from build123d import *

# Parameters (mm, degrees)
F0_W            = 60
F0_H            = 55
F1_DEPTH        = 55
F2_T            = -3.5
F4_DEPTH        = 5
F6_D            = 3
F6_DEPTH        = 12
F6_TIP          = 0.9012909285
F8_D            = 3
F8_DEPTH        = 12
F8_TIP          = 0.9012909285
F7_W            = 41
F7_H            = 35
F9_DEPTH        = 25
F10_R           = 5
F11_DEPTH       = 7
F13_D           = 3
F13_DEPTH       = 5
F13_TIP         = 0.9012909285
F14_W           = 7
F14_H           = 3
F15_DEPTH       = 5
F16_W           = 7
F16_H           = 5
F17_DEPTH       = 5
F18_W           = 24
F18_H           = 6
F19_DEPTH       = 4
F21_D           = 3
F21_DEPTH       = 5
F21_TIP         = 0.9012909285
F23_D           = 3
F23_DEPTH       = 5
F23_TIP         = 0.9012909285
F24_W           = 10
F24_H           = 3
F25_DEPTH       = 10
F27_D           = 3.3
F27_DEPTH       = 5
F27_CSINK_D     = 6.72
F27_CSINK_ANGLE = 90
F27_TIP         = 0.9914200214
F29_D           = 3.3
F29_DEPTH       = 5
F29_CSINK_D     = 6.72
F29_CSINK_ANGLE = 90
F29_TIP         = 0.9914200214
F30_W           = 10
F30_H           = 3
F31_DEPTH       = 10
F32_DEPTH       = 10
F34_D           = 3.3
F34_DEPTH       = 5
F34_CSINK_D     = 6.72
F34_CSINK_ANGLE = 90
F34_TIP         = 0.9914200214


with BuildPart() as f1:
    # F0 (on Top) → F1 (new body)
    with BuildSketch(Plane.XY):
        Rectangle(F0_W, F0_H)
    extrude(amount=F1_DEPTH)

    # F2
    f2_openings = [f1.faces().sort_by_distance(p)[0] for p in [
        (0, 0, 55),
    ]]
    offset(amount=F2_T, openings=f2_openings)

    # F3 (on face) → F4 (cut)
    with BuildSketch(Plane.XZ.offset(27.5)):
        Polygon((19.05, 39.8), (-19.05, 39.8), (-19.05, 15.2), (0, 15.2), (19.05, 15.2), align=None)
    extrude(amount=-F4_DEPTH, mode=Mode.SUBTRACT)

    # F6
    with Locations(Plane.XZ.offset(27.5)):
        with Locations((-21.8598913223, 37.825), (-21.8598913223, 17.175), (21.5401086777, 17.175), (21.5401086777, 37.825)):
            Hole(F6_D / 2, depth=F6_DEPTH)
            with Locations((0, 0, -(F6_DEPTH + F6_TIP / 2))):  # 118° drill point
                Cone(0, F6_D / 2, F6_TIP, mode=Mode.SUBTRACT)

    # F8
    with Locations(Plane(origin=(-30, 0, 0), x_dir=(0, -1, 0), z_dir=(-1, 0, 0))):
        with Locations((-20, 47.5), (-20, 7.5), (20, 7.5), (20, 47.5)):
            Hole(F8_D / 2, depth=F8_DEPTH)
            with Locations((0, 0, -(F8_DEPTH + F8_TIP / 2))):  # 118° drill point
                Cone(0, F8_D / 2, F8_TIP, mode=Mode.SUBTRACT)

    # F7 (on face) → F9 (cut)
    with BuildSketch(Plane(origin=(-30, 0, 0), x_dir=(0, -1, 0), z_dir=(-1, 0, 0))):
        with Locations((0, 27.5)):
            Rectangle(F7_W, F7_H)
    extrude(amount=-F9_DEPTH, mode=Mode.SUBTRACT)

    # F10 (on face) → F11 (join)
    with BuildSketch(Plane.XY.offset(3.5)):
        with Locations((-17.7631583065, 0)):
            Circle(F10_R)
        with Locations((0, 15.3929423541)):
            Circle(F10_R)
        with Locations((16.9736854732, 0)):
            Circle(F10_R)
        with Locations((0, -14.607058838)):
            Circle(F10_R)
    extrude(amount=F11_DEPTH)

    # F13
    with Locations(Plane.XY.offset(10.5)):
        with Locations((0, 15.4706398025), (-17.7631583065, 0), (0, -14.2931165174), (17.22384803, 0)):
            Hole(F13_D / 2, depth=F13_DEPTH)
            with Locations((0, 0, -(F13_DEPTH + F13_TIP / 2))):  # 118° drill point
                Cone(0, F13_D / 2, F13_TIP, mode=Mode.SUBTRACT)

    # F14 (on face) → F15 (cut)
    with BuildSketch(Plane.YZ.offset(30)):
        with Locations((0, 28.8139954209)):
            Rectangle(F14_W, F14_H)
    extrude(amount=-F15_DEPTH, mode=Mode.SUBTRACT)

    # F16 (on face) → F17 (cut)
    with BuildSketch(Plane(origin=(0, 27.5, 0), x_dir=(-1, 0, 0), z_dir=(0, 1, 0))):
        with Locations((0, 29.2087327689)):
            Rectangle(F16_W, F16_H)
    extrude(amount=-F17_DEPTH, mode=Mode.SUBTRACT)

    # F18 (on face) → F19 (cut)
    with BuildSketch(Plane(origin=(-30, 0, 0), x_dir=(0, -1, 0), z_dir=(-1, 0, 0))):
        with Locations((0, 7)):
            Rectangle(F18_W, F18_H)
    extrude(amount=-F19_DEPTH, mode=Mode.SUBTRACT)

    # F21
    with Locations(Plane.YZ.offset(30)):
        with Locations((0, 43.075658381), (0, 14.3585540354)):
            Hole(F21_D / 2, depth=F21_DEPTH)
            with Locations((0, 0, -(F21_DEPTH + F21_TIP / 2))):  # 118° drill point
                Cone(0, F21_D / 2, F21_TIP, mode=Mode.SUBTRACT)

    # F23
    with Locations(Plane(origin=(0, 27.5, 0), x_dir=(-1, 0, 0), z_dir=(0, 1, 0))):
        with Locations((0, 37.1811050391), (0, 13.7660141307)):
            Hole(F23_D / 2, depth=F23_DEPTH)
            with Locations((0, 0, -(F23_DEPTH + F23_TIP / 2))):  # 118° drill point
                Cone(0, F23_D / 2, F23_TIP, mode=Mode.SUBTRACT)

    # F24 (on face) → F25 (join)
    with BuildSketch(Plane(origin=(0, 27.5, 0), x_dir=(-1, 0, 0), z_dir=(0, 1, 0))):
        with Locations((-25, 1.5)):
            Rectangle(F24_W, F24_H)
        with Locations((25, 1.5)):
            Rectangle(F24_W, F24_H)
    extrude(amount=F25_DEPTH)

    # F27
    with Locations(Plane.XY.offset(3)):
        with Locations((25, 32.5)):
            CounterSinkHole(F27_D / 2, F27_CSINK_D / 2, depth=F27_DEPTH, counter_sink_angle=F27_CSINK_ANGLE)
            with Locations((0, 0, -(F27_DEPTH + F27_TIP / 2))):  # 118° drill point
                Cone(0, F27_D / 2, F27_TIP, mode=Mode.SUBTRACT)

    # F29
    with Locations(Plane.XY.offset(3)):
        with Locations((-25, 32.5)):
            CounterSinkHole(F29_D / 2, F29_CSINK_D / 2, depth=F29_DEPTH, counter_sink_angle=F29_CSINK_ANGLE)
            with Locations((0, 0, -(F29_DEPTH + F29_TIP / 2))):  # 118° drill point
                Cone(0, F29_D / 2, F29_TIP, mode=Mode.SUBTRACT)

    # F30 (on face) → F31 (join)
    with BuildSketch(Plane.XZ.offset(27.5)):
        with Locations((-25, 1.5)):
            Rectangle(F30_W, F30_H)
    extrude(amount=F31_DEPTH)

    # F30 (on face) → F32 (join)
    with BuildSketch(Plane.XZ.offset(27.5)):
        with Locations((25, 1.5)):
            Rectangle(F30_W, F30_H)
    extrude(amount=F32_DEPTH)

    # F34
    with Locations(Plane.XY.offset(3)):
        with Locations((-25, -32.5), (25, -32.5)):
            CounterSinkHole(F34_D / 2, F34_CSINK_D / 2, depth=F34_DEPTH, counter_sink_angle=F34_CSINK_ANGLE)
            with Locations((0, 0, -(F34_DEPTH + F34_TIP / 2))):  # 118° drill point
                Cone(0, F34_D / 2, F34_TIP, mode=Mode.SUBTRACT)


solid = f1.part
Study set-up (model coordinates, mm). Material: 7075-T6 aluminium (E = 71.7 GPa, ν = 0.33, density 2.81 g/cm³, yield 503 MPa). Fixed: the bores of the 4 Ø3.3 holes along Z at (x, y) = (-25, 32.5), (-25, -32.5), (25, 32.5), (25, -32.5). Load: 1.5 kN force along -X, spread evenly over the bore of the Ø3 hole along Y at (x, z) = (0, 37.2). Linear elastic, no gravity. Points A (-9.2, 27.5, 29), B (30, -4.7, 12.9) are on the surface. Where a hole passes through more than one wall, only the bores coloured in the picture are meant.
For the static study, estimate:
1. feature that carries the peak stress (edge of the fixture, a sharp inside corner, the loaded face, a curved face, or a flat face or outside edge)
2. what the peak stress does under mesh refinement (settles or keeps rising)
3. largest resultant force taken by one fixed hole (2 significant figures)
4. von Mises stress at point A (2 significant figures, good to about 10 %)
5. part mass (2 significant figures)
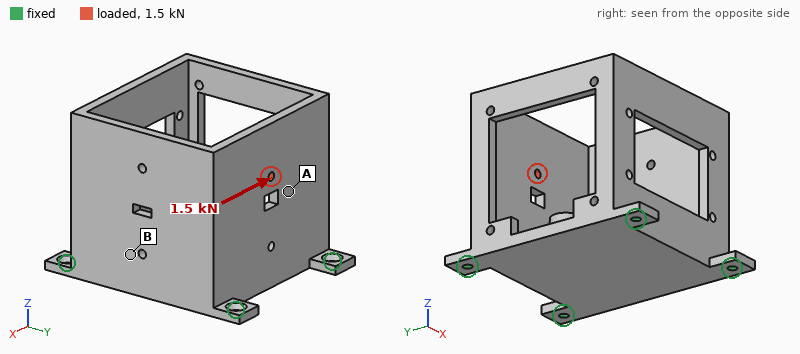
edge of the fixture
keeps rising
1.2 kN
20 MPa
120 g
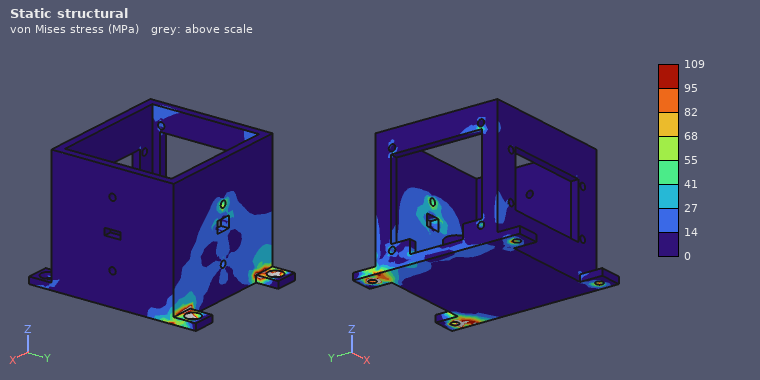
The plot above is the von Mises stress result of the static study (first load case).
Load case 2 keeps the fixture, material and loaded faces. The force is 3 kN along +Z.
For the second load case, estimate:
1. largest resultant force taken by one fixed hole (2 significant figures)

1.5 kN
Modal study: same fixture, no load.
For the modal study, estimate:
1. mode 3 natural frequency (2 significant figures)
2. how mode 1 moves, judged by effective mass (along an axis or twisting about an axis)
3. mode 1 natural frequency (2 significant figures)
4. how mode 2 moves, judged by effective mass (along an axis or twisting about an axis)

3300 Hz
along Y
2000 Hz
along X
